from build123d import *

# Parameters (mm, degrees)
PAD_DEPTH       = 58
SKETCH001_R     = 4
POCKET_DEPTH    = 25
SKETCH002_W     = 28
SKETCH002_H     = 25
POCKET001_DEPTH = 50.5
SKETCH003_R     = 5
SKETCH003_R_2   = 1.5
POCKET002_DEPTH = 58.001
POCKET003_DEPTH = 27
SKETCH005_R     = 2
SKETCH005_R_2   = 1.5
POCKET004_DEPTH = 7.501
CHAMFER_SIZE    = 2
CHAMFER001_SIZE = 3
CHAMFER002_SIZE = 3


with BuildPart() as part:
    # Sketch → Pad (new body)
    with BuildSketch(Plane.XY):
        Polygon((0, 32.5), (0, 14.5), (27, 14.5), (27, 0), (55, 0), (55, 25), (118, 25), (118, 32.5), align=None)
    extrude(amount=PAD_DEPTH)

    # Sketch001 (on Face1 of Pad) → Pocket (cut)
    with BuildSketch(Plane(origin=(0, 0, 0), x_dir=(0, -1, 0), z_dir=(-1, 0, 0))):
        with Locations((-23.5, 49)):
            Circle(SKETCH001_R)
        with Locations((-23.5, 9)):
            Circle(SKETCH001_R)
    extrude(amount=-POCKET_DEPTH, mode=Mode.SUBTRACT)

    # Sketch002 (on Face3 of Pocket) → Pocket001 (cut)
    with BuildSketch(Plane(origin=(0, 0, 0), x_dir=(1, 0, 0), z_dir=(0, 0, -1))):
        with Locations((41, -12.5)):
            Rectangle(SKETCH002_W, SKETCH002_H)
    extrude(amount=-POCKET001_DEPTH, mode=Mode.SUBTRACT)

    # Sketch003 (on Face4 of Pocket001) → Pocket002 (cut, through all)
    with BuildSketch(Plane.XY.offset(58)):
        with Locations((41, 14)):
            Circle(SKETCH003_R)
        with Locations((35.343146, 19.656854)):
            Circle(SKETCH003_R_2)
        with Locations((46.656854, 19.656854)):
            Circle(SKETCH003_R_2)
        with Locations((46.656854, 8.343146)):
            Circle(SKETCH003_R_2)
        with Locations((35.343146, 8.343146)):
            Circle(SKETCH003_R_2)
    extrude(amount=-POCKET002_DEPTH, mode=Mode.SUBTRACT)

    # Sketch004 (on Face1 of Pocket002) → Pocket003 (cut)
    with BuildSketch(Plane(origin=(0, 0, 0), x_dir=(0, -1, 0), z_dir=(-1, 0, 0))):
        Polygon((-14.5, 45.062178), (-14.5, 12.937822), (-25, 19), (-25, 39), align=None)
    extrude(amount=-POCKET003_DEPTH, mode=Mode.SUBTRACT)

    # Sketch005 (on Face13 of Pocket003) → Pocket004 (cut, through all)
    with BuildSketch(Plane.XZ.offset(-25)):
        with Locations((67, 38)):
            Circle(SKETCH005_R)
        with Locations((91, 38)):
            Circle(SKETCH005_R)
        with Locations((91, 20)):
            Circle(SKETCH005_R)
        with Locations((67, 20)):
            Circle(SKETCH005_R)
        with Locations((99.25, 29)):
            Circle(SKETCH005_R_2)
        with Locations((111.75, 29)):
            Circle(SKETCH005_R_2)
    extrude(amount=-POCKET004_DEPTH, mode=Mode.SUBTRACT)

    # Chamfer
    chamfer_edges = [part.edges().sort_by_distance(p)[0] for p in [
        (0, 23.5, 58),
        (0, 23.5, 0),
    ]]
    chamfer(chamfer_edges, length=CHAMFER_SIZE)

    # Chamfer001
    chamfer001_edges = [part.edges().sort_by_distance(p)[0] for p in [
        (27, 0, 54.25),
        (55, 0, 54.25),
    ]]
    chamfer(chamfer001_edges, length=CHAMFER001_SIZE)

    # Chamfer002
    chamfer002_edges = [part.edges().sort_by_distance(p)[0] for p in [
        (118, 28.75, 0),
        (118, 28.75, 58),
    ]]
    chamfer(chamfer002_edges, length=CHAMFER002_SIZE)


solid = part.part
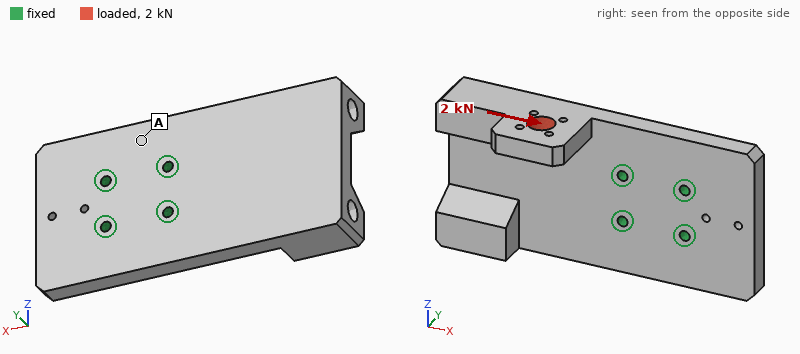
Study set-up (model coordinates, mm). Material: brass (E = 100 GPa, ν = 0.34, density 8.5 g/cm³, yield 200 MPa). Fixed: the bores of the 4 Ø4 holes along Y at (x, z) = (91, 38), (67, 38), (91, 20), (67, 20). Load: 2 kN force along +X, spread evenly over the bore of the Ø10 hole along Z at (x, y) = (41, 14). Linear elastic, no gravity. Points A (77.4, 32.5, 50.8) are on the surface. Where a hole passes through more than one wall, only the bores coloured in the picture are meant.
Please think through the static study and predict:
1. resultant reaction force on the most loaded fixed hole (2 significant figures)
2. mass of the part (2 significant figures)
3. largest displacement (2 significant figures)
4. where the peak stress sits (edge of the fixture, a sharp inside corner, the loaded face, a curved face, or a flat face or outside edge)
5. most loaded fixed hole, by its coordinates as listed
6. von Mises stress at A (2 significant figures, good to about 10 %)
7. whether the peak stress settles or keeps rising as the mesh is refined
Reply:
1.8 kN
520 g
0.25 mm
edge of the fixture
(67, 38)
12 MPa
keeps rising
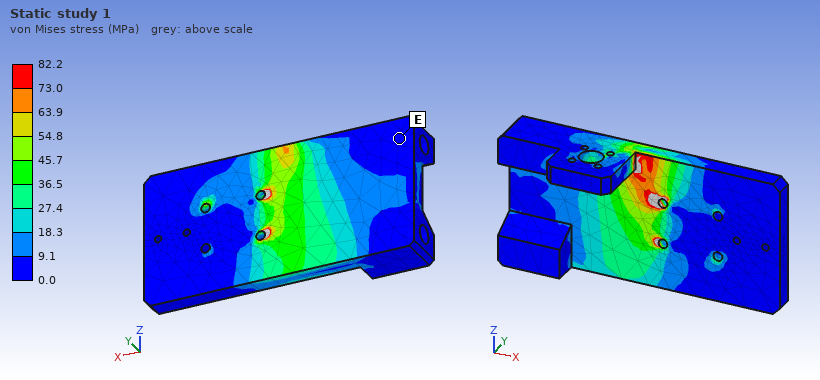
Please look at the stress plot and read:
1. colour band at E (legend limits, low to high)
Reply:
0.0 to 9.1 MPa
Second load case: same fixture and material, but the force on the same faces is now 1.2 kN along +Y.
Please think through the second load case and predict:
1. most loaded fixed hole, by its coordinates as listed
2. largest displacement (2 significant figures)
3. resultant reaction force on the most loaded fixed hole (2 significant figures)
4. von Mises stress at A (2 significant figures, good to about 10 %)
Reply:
(67, 38)
0.21 mm
1.9 kN
29 MPa
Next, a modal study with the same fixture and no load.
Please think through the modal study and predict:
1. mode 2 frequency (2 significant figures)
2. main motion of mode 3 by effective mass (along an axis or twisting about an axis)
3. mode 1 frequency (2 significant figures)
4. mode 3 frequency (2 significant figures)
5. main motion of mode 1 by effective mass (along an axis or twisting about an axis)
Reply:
1600 Hz
along Z
750 Hz
3000 Hz
along Y
